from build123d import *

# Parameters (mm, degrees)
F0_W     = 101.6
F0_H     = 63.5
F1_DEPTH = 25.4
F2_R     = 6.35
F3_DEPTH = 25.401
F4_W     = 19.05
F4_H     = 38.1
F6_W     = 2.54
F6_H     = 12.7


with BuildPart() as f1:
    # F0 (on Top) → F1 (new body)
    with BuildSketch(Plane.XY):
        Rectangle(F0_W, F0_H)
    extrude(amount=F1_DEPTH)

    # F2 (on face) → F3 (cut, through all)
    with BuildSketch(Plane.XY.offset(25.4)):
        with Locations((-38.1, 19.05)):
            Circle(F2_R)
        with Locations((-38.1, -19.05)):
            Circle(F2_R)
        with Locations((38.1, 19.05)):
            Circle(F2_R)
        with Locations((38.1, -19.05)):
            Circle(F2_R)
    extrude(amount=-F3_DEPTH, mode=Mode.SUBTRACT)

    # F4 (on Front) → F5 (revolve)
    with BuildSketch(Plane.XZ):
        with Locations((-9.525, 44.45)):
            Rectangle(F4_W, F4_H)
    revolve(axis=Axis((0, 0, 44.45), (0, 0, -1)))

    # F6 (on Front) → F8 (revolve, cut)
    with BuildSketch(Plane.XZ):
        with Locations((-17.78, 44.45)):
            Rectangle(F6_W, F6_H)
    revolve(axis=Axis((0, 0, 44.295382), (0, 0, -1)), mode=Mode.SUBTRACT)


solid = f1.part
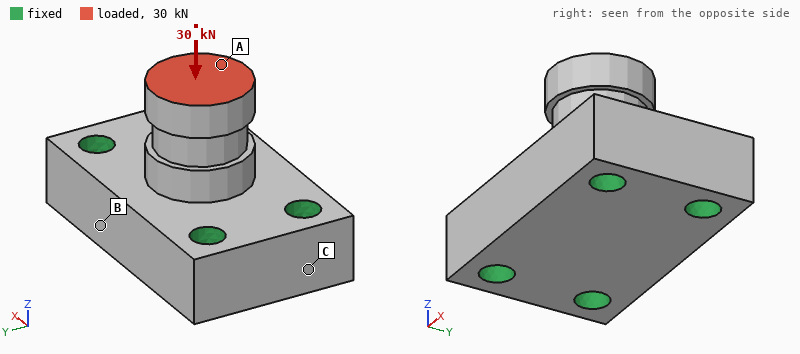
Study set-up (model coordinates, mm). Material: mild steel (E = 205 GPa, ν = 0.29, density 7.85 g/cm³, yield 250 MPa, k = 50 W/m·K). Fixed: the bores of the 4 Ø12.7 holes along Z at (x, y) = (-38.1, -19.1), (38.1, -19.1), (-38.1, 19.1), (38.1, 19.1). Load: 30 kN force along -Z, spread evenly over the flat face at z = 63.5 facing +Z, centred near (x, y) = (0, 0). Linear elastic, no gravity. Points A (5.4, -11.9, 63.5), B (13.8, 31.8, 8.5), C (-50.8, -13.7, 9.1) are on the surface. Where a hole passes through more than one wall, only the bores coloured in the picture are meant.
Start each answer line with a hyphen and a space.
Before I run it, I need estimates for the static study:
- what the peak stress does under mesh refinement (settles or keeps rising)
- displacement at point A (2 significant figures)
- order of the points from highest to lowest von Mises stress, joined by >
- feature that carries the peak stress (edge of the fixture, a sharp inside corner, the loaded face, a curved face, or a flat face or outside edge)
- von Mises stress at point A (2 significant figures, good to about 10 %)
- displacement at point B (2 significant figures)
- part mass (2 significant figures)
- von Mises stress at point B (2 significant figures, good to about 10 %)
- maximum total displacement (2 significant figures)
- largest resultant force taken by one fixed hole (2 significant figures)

- keeps rising
- 11 µm
- A > B > C
- edge of the fixture
- 30 MPa
- 3.4 µm
- 1.5 kg
- 13 MPa
- 12 µm
- 7.7 kN
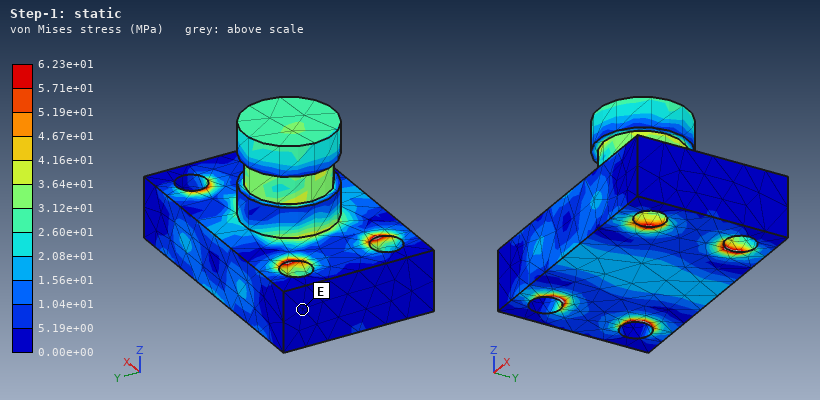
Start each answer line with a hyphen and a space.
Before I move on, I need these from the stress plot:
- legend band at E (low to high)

- 0.00e+00 to 5.19e+00 MPa
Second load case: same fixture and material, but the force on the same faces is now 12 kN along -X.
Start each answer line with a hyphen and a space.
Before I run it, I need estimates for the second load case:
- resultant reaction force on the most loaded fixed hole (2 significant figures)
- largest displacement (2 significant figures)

- 6.0 kN
- 35 µm
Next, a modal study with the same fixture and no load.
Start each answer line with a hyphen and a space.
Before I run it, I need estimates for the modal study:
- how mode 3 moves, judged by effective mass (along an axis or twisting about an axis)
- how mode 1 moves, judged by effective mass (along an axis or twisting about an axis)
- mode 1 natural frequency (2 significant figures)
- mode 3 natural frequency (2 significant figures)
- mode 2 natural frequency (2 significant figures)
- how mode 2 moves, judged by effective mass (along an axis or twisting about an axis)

- along Z
- along Y
- 8000 Hz
- 13 kHz
- 9400 Hz
- along X
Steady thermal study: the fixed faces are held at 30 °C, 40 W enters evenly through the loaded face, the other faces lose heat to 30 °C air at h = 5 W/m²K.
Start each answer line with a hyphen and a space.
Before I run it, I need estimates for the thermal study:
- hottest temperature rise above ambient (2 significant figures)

- 41 K
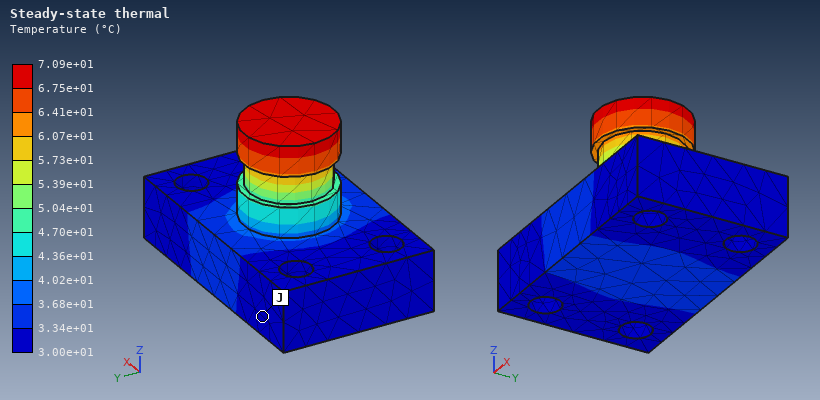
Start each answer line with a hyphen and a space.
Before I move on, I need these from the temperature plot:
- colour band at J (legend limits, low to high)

- 3.00e+01 to 3.34e+01 °C
